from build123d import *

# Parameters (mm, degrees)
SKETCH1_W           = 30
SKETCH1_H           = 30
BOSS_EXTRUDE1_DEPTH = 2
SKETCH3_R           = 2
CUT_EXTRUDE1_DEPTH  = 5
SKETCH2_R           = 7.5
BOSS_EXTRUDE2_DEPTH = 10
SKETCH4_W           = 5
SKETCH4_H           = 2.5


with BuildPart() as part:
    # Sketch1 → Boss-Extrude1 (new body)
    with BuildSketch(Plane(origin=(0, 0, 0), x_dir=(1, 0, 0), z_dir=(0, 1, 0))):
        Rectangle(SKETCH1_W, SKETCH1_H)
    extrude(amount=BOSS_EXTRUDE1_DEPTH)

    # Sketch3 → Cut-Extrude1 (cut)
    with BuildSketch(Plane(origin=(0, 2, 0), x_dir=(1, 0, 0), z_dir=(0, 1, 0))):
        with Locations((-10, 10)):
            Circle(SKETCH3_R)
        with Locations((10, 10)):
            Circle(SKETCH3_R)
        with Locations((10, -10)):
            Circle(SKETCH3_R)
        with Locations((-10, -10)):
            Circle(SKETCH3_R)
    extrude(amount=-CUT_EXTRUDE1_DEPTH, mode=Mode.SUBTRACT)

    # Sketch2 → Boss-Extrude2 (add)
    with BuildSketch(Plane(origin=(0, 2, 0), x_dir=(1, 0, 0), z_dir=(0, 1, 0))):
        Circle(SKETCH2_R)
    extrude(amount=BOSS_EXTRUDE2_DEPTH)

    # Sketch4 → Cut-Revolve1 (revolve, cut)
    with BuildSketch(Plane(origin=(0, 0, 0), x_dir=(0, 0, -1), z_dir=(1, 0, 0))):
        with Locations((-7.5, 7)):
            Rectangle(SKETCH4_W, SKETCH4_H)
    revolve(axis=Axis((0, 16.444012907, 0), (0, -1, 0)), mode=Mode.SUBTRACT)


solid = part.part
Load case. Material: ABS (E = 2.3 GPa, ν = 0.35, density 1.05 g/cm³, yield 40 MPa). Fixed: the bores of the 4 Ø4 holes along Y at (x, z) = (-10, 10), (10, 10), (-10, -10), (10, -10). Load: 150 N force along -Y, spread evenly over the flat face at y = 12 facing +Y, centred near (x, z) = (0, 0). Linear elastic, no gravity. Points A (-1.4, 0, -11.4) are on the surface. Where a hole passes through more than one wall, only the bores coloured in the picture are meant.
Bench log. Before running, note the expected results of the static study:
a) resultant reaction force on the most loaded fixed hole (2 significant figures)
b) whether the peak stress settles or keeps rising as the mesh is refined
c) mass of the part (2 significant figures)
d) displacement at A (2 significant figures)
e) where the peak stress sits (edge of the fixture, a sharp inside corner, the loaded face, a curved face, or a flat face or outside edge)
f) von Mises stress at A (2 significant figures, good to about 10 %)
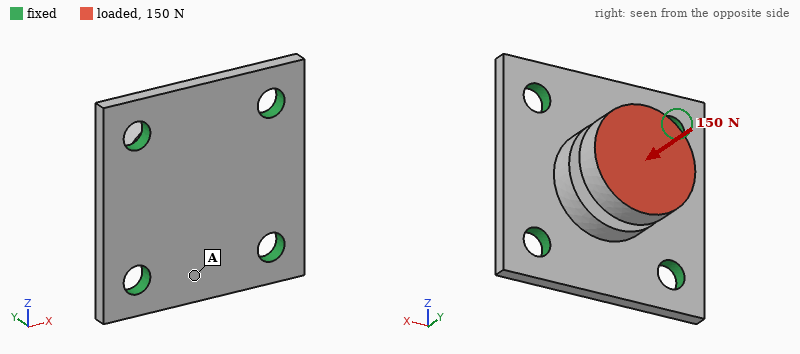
41 N
keeps rising
3.4 g
36 µm
edge of the fixture
3.8 MPa
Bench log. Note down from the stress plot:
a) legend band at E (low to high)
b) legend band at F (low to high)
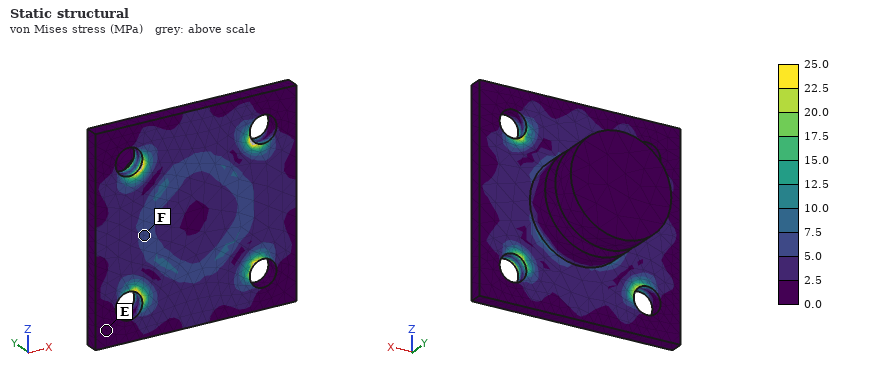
0.0 to 2.5 MPa
5.0 to 7.5 MPa
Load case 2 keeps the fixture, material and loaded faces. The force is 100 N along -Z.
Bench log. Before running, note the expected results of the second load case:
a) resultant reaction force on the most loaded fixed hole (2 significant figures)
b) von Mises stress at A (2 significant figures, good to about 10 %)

44 N
5.0 MPa
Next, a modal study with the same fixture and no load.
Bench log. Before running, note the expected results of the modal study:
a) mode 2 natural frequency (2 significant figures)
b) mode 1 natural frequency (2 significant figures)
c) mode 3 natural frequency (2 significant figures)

5000 Hz
5000 Hz
5000 Hz
